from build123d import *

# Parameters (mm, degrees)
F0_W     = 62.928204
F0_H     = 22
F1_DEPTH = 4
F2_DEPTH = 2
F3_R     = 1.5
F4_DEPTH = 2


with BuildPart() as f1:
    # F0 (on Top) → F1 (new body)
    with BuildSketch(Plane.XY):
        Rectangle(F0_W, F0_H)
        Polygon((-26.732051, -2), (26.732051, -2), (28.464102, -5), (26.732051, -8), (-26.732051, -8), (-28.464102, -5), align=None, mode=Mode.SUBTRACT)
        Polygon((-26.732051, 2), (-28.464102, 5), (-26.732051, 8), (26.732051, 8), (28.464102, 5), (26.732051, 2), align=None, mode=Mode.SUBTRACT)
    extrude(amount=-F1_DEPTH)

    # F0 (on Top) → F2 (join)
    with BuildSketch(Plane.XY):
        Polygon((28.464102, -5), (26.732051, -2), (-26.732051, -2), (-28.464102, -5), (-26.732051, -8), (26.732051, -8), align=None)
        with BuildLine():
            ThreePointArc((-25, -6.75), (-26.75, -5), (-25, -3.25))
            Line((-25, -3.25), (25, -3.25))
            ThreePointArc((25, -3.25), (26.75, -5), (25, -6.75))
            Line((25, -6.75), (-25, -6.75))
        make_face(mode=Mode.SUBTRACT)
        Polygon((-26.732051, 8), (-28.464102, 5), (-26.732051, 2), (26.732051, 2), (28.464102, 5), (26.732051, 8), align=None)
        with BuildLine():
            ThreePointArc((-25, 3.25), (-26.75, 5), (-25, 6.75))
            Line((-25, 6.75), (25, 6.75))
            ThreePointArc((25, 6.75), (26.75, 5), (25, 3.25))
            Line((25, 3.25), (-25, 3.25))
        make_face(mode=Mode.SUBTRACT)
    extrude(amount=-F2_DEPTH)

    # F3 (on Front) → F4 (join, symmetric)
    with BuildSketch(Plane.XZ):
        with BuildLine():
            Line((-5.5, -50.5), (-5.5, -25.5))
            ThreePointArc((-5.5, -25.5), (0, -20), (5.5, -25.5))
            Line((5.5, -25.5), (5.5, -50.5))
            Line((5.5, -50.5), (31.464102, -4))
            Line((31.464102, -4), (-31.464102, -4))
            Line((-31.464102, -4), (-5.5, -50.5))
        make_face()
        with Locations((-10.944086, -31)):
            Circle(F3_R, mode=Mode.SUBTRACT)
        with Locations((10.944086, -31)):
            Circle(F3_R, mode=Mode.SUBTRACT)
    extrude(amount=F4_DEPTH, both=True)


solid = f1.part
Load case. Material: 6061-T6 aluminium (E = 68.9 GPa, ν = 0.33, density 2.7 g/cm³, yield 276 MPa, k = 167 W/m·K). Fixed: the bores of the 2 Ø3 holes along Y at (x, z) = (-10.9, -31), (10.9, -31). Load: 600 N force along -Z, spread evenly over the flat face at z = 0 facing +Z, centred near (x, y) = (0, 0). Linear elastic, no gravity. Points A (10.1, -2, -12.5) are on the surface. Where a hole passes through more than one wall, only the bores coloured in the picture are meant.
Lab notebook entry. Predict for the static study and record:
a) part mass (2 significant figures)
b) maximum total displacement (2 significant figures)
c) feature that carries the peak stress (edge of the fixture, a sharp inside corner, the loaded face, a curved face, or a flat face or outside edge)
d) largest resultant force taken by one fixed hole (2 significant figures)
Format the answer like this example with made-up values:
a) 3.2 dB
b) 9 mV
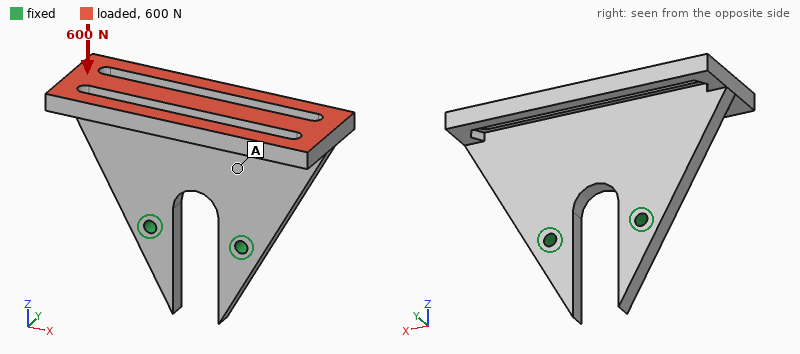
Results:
a) 24 g
b) 0.13 mm
c) a curved face
d) 310 N
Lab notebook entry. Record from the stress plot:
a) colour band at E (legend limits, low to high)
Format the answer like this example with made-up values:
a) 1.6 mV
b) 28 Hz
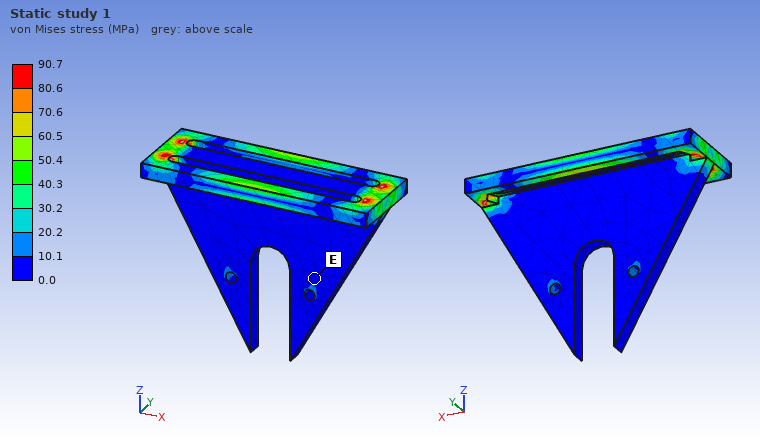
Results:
a) 0.0 to 10.1 MPa
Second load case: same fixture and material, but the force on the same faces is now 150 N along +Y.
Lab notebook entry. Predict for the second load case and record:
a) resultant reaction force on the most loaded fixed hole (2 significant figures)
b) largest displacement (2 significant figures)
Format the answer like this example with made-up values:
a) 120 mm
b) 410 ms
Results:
a) 75 N
b) 0.17 mm
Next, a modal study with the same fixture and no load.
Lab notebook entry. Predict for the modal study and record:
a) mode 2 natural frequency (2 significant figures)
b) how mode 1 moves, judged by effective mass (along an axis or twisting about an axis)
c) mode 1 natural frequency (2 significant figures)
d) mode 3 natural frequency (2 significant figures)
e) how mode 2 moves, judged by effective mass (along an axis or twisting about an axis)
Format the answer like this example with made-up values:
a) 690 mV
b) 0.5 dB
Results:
a) 2300 Hz
b) along Y
c) 1500 Hz
d) 3600 Hz
e) twisting about Z
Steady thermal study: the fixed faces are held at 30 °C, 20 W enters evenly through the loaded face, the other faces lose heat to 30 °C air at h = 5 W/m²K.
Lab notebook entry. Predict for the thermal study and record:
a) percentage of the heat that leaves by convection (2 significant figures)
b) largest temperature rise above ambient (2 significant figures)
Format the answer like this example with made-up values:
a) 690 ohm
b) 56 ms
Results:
a) 3.3 %
b) 49 K
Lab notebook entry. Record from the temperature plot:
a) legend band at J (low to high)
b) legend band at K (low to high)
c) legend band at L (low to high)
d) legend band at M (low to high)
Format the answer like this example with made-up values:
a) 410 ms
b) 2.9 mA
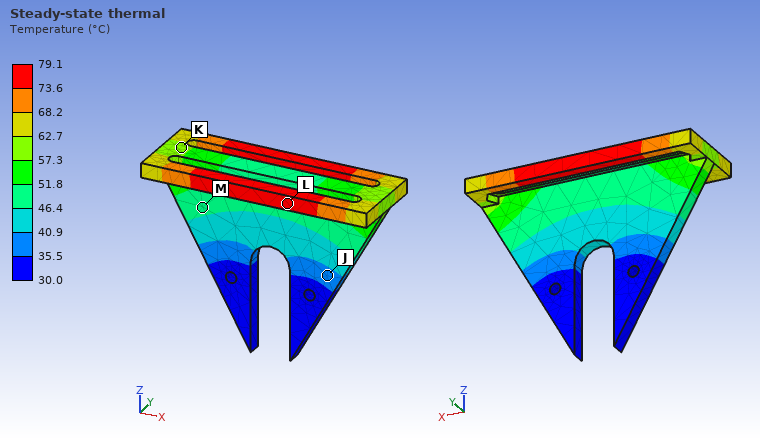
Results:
a) 35.5 to 40.9 °C
b) 57.3 to 62.7 °C
c) 73.6 to 79.1 °C
d) 46.4 to 51.8 °C
